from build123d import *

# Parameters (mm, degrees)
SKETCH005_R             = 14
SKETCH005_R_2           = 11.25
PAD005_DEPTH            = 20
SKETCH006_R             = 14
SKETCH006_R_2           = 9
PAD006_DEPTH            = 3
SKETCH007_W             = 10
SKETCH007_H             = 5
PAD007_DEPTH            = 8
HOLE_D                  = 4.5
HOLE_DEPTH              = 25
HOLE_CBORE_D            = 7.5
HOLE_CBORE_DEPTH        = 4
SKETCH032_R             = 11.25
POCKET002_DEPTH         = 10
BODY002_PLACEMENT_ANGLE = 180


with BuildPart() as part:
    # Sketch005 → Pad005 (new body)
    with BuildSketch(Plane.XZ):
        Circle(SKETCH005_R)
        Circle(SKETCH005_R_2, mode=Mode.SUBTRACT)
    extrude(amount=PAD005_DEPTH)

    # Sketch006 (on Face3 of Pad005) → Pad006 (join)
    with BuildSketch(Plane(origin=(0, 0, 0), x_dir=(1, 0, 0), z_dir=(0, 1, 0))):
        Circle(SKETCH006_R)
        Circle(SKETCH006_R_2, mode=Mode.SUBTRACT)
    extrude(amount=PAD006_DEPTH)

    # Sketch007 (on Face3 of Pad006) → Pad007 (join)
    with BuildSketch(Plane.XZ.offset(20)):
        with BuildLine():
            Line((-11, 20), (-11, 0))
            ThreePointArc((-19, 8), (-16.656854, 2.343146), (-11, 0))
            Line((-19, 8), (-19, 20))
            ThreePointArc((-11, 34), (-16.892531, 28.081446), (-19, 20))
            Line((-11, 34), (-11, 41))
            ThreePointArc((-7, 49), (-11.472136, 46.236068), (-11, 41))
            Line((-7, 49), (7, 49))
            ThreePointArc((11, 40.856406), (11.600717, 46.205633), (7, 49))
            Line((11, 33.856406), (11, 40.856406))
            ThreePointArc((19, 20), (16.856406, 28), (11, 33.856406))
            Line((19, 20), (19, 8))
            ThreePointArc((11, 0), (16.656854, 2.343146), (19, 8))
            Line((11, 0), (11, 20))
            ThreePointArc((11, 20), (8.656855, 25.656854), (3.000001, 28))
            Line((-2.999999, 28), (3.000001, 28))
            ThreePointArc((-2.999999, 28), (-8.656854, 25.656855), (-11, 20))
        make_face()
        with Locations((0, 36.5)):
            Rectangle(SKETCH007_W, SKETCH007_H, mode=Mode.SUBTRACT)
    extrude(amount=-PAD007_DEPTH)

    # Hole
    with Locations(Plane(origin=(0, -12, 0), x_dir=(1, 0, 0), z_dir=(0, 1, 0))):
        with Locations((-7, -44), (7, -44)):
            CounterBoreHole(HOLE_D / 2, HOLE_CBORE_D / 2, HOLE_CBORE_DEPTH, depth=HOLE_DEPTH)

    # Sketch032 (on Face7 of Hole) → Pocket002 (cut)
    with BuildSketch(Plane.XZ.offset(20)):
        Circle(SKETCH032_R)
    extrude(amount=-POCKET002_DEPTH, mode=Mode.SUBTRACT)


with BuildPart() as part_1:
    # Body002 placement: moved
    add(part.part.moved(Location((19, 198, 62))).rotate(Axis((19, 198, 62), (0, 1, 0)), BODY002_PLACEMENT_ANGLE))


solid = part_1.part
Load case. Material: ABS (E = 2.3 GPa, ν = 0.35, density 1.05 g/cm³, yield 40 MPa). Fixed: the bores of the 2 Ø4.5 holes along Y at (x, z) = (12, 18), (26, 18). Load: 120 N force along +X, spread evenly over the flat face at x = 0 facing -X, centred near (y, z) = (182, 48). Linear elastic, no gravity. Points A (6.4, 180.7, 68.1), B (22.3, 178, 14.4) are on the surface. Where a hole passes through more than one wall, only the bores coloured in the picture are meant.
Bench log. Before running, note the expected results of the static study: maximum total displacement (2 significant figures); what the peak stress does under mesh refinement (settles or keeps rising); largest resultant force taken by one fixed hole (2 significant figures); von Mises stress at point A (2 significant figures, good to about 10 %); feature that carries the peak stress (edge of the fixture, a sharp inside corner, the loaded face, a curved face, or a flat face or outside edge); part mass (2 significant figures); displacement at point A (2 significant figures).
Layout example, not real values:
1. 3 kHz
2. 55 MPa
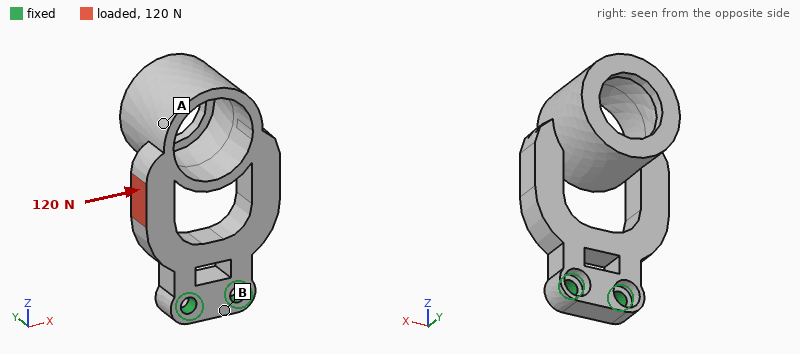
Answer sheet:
1. 0.75 mm
2. keeps rising
3. 200 N
4. 2.1 MPa
5. edge of the fixture
6. 12 g
7. 0.70 mm
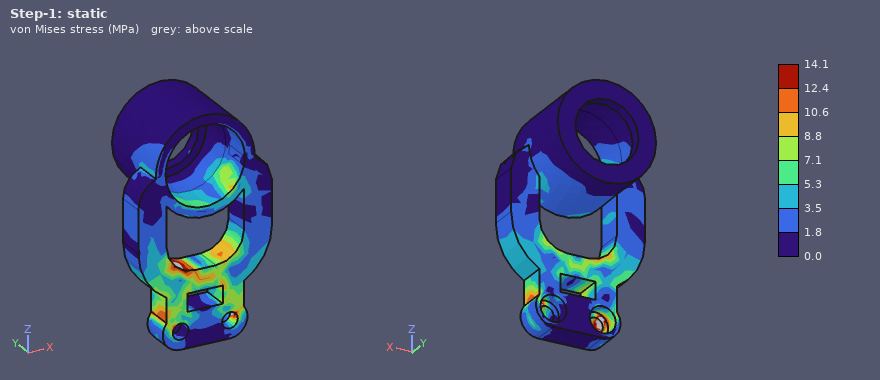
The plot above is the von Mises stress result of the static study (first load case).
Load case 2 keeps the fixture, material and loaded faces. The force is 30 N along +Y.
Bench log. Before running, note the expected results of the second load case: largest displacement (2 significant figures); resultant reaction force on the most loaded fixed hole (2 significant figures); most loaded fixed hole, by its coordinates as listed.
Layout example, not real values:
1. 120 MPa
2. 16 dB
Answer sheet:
1. 0.87 mm
2. 49 N
3. (12, 18)
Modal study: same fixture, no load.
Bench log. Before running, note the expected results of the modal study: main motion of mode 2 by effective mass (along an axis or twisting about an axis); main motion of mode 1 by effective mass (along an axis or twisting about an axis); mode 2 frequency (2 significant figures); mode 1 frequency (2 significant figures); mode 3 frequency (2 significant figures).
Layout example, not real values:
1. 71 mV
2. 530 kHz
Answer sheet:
1. along X
2. along Y
3. 650 Hz
4. 320 Hz
5. 950 Hz
